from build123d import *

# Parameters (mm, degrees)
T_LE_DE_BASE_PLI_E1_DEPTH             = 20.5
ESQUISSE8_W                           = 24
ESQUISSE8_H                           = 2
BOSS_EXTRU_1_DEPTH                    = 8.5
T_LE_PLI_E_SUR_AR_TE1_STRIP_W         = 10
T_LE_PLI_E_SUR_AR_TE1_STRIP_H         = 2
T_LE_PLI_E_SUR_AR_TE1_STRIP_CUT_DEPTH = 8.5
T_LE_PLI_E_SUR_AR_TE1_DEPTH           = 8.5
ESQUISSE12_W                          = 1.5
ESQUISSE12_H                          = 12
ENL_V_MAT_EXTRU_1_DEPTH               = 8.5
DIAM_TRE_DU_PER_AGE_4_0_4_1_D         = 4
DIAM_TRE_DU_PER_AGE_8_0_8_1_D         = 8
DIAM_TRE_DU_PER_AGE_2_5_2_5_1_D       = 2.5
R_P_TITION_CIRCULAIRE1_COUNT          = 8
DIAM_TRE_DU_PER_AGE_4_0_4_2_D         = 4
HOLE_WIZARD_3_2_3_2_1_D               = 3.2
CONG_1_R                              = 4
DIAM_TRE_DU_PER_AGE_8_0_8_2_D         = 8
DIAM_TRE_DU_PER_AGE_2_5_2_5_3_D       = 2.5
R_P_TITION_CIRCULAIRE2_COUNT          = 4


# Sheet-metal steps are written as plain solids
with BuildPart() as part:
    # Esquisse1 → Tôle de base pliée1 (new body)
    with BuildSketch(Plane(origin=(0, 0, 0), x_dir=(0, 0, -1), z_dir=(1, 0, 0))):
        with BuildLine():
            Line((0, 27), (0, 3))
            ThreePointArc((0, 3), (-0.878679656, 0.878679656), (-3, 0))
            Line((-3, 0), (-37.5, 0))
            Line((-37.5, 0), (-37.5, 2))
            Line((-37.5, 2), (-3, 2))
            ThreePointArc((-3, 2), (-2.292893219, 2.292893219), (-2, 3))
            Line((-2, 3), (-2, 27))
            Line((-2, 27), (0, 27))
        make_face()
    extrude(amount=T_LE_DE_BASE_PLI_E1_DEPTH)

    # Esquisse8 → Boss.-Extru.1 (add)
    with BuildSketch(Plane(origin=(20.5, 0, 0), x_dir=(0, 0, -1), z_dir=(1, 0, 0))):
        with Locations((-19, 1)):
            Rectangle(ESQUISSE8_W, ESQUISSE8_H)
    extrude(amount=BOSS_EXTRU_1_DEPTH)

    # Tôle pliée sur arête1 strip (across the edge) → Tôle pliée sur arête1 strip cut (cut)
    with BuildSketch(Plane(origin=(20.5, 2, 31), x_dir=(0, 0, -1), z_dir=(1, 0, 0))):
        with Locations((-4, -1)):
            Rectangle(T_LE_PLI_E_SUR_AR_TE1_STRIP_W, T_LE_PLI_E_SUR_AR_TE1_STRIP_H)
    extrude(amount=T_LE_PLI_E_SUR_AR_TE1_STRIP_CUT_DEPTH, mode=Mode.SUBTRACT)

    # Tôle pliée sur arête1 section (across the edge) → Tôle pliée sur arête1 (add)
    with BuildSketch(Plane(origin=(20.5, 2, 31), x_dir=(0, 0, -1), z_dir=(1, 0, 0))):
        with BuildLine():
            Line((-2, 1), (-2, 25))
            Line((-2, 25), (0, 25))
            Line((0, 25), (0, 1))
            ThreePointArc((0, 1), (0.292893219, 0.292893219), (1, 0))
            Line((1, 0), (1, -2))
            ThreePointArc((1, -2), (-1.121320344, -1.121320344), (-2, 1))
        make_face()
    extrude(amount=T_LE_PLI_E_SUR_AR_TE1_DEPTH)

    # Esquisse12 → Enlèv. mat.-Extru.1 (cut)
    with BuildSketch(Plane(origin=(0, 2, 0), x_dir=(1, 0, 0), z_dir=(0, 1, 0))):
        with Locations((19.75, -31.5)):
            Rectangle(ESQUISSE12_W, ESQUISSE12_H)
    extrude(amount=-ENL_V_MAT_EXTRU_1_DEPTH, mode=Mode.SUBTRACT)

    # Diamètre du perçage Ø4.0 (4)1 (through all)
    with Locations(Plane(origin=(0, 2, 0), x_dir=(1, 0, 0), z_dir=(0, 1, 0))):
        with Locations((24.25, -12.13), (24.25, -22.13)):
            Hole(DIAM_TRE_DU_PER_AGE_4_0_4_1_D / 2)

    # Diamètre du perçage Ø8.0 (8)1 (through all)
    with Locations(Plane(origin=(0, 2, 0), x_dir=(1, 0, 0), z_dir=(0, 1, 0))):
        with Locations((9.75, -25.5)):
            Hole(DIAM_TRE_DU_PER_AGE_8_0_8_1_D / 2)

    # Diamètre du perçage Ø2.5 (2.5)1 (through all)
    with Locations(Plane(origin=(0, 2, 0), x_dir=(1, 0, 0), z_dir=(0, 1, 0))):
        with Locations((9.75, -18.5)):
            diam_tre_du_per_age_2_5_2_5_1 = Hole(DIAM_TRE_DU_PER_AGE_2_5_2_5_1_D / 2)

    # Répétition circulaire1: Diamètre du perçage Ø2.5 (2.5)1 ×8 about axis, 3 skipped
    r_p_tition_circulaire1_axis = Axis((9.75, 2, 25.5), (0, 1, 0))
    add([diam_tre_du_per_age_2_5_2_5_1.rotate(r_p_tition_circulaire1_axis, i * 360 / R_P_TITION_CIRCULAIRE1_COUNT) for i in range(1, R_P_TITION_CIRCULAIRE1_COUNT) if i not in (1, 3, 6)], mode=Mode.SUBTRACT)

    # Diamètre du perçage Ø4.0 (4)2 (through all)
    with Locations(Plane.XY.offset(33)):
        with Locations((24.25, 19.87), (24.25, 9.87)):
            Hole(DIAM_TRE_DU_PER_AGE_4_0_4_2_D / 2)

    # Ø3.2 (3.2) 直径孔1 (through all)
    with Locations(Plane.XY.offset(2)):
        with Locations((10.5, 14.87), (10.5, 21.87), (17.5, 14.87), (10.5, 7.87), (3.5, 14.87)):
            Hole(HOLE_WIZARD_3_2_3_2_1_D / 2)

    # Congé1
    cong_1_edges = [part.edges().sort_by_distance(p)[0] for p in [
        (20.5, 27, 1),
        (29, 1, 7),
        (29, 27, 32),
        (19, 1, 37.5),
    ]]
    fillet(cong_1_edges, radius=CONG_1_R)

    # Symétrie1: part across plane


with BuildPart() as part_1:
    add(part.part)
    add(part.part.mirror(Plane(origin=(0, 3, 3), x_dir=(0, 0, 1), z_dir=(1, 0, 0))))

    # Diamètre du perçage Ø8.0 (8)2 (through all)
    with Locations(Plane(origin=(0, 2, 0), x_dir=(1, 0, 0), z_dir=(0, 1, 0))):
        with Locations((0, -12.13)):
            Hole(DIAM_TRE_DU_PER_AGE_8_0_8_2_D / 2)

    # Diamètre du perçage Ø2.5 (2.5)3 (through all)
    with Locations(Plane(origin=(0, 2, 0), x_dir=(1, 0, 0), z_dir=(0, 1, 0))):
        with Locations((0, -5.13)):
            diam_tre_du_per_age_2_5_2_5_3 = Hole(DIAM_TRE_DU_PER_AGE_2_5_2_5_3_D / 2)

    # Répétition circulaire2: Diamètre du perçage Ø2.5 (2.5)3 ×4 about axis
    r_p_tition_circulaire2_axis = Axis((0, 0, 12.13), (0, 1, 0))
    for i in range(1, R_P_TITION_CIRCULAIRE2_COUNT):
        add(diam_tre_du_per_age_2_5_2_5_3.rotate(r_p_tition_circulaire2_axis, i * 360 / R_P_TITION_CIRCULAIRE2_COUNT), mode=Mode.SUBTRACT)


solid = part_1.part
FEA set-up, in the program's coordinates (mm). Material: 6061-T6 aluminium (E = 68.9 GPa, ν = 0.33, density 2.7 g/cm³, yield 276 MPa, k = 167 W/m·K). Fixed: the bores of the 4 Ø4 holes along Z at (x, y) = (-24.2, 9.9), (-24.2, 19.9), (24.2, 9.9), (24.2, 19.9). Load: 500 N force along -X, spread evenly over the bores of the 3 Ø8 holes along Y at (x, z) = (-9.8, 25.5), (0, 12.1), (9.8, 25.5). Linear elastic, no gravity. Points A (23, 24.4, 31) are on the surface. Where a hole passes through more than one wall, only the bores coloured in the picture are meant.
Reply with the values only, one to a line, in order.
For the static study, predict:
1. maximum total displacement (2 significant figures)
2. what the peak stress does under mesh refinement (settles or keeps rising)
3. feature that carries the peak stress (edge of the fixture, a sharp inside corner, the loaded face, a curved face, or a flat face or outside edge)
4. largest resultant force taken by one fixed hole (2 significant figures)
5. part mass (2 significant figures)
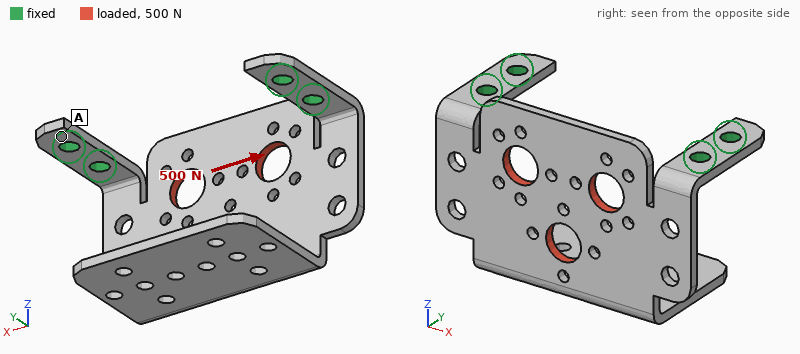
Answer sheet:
0.14 mm
keeps rising
edge of the fixture
310 N
16 g
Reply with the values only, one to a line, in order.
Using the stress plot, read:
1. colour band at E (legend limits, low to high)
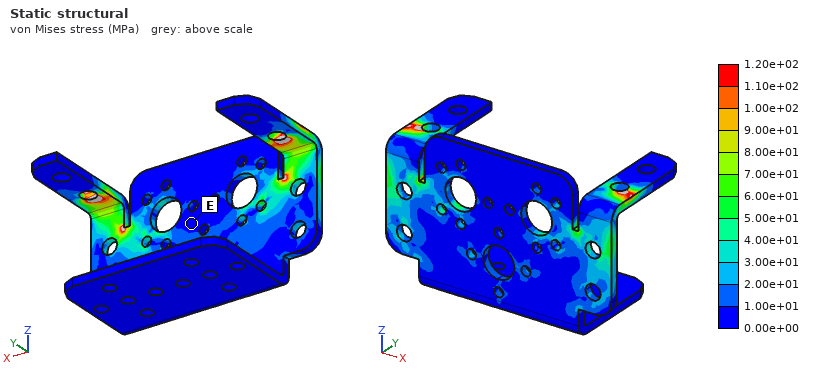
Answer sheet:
0.00e+00 to 1.00e+01 MPa
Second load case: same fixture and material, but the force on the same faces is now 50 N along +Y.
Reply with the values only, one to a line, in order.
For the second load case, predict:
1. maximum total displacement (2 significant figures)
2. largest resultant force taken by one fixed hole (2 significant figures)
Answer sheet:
0.34 mm
25 N
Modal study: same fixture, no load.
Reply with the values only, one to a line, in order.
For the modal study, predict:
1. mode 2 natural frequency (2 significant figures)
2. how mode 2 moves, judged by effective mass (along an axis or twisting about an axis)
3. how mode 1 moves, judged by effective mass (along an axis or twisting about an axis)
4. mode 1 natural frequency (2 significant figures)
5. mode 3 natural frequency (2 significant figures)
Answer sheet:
1100 Hz
along X
along Y
380 Hz
1500 Hz
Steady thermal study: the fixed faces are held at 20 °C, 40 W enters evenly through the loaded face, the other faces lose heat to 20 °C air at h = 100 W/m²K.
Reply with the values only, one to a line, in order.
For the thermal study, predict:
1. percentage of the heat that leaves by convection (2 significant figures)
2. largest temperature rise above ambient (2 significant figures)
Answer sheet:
70 %
72 K
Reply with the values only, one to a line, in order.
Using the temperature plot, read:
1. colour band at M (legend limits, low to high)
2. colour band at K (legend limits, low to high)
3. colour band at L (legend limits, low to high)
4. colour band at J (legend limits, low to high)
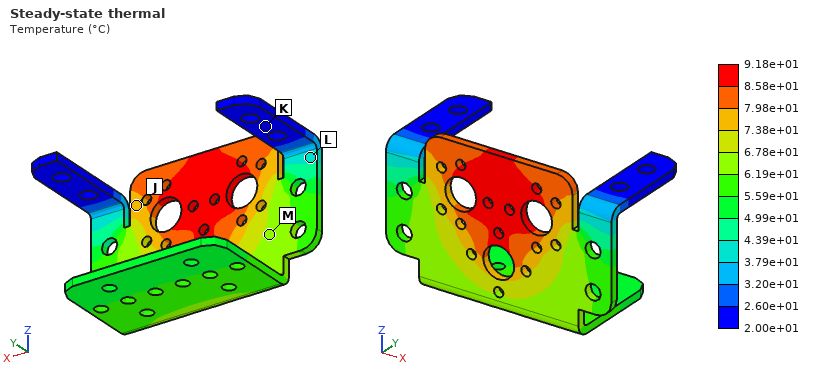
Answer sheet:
6.19e+01 to 6.78e+01 °C
2.00e+01 to 2.60e+01 °C
3.79e+01 to 4.39e+01 °C
7.38e+01 to 7.98e+01 °C
